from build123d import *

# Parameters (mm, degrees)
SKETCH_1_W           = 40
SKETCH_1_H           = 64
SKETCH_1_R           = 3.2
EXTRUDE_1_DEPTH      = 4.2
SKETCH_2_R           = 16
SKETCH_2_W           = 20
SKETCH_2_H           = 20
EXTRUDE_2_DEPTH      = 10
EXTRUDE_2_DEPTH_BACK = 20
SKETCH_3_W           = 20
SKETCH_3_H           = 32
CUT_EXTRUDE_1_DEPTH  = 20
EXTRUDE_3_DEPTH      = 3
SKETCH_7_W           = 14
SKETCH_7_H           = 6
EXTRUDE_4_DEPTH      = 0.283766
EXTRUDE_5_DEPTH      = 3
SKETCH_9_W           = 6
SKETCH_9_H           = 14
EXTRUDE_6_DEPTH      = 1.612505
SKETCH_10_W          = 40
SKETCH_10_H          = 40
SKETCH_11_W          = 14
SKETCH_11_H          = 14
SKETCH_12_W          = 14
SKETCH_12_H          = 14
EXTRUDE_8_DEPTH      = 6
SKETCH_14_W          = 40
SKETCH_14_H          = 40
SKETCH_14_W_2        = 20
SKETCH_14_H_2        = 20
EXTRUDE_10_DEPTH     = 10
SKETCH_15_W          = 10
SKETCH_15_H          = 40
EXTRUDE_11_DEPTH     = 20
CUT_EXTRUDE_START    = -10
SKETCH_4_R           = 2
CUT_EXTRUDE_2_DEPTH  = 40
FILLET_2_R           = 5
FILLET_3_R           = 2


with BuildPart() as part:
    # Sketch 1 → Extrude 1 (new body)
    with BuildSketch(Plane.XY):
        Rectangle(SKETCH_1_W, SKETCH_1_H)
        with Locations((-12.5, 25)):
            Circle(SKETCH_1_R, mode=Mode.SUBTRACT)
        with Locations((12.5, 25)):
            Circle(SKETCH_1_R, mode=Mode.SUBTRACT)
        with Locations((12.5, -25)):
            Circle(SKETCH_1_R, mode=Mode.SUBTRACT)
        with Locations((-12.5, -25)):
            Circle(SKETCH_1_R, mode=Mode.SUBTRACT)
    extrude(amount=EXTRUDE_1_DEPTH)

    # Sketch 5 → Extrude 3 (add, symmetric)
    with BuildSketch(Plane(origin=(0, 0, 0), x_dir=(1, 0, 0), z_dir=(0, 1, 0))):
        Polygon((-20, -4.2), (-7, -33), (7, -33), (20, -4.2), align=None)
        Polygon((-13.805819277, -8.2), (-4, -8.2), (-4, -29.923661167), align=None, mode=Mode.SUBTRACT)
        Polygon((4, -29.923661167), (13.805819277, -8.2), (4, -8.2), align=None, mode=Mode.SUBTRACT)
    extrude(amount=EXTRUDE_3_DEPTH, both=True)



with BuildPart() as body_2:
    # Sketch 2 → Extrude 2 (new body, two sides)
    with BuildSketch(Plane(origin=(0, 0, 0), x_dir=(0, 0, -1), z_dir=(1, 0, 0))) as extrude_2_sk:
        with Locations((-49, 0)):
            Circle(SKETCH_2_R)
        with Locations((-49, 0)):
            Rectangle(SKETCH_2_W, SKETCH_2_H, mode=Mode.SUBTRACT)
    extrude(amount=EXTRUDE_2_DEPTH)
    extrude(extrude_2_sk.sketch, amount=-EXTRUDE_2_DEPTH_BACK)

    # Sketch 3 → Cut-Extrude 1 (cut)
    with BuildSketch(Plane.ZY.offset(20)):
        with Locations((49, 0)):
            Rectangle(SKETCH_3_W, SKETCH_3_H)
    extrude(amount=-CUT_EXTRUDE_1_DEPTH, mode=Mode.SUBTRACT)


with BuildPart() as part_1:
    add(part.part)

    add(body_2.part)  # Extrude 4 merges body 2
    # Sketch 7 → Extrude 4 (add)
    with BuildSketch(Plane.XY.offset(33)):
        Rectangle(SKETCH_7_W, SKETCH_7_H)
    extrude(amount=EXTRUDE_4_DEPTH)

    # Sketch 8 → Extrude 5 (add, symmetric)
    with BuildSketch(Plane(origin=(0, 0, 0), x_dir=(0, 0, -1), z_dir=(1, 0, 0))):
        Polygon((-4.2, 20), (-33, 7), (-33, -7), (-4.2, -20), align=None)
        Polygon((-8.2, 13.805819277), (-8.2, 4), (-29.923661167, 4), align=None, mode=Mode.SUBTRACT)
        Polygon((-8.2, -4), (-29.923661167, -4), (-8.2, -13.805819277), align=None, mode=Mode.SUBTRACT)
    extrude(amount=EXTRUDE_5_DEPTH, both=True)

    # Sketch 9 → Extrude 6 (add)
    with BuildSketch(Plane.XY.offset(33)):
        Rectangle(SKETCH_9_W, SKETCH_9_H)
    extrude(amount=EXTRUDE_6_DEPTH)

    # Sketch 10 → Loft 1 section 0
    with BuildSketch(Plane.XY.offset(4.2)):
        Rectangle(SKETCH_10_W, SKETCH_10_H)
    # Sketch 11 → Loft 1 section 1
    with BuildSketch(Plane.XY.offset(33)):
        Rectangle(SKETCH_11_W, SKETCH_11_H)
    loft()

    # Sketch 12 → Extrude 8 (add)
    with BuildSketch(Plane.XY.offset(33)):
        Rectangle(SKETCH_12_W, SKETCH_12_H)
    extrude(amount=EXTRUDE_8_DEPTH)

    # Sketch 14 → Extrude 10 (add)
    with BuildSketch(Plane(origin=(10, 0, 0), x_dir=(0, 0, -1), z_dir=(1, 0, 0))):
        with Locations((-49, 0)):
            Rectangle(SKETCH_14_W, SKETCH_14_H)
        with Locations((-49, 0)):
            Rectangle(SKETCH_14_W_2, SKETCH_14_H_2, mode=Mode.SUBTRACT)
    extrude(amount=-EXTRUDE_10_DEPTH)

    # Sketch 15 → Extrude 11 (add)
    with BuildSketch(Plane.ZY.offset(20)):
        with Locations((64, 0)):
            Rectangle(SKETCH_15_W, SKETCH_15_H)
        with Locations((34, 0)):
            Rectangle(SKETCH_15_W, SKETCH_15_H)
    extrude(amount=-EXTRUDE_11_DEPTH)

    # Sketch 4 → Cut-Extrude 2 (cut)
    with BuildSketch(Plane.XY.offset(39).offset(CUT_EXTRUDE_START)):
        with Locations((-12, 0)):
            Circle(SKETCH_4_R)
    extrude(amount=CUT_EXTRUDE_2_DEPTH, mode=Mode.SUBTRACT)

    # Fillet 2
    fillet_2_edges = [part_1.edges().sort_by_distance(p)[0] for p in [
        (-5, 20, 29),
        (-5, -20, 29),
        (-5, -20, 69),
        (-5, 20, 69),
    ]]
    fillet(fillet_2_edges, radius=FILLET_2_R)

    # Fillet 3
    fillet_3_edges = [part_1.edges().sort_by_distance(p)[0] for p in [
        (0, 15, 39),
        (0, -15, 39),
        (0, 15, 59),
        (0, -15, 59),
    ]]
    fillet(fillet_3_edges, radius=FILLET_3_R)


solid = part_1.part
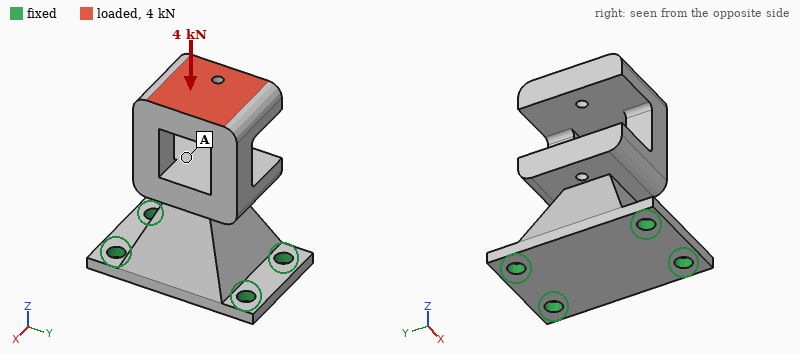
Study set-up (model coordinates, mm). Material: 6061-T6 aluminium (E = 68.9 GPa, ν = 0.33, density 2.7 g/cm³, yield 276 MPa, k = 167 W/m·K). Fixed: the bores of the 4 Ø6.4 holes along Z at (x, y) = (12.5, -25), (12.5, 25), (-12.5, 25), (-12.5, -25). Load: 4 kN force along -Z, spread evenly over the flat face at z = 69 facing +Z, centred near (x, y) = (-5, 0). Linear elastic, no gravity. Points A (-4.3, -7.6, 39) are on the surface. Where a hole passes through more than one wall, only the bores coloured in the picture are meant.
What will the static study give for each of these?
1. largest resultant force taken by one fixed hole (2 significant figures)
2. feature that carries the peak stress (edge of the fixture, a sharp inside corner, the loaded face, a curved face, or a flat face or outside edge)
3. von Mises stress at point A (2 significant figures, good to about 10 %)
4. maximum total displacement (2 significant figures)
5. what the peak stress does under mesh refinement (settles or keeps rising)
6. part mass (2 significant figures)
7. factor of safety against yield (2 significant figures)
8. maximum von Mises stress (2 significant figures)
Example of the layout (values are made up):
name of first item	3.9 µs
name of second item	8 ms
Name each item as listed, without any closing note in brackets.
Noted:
largest resultant force taken by one fixed hole	1.6 kN
feature that carries the peak stress	a curved face
von Mises stress at point A	27 MPa
maximum total displacement	0.38 mm
what the peak stress does under mesh refinement	settles
part mass	160 g
factor of safety against yield	0.94
maximum von Mises stress	290 MPa
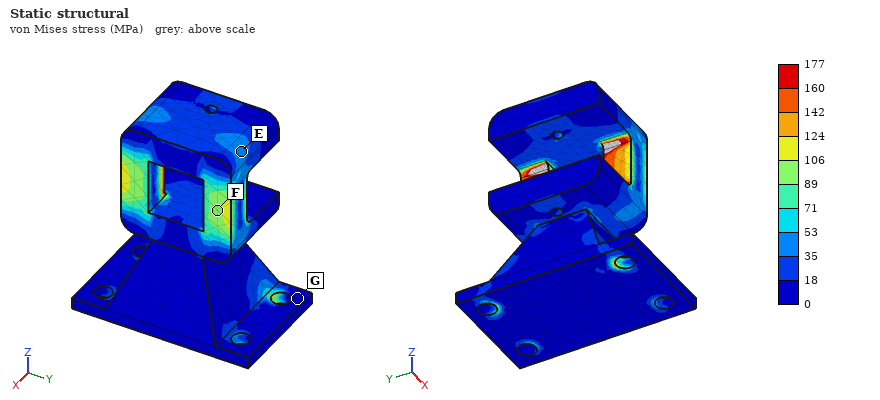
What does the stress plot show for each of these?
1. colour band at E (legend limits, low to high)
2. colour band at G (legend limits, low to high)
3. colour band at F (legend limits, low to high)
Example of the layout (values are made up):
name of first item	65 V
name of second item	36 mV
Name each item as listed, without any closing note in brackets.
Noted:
colour band at E	35 to 53 MPa
colour band at G	0 to 18 MPa
colour band at F	89 to 106 MPa
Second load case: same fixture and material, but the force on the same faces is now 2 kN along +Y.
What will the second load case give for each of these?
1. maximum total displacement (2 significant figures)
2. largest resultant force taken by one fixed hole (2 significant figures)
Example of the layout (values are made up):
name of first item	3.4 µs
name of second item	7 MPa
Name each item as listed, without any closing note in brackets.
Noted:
maximum total displacement	0.27 mm
largest resultant force taken by one fixed hole	1.7 kN
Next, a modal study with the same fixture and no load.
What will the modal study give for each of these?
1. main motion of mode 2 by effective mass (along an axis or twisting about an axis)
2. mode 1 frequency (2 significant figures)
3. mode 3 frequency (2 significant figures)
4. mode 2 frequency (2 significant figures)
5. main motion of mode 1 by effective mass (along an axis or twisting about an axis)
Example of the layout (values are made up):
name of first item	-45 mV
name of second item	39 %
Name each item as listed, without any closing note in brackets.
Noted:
main motion of mode 2 by effective mass	along Y
mode 1 frequency	1900 Hz
mode 3 frequency	4800 Hz
mode 2 frequency	2600 Hz
main motion of mode 1 by effective mass	along X
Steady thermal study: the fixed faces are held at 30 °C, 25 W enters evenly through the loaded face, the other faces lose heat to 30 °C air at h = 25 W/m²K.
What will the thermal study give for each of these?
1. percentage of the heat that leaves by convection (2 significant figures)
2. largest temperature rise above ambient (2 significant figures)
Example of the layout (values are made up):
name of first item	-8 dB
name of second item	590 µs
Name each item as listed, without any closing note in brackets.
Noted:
percentage of the heat that leaves by convection	17 %
largest temperature rise above ambient	34 K
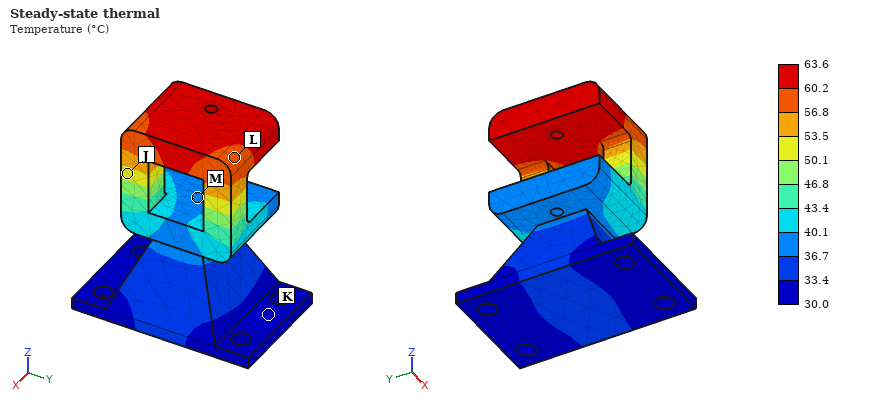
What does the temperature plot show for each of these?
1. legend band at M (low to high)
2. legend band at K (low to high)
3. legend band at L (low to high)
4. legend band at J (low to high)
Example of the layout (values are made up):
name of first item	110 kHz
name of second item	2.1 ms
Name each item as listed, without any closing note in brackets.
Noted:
legend band at M	36.7 to 40.1 °C
legend band at K	30.0 to 33.4 °C
legend band at L	56.8 to 60.2 °C
legend band at J	50.1 to 53.5 °C
